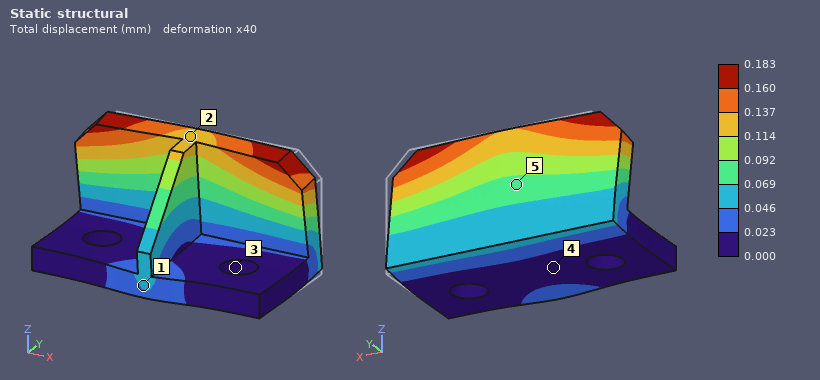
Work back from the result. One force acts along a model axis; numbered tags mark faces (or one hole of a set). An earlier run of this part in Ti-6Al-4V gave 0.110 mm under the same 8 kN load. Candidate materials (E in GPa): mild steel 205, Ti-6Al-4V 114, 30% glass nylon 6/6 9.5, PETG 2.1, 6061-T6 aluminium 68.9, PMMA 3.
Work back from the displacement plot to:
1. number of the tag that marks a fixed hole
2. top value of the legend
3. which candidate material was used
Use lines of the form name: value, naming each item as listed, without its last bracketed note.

number of the tag that marks a fixed hole: 3
top value of the legend: 0.183 mm
which candidate material was used: 6061-T6 aluminium
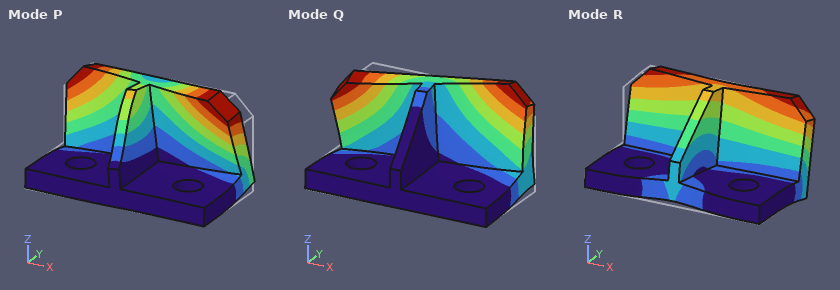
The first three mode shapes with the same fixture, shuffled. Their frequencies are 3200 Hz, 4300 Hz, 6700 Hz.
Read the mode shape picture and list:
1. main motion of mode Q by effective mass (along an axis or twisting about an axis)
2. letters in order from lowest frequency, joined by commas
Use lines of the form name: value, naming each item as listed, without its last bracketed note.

main motion of mode Q by effective mass: along X
letters in order from lowest frequency, joined by commas: R, P, Q
